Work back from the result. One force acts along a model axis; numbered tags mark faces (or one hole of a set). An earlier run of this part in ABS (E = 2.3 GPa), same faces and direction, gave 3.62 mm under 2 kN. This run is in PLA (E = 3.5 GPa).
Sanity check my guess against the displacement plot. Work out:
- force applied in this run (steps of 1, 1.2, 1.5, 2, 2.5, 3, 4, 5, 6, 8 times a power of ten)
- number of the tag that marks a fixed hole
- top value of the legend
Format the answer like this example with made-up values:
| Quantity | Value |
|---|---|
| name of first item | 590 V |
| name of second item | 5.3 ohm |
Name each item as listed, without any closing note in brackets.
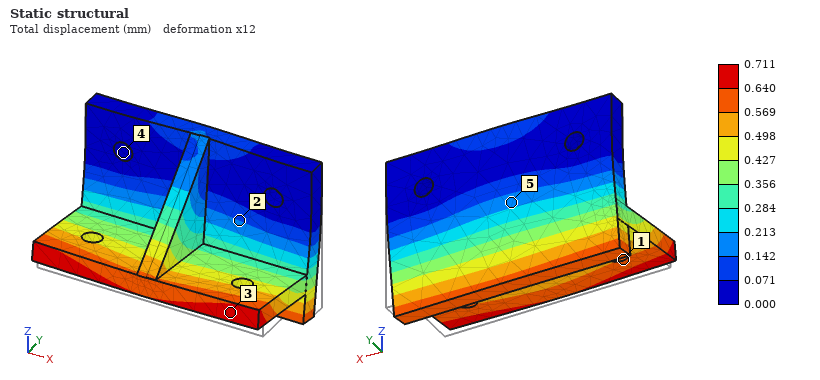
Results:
| Quantity | Value |
|---|---|
| force applied in this run | 600 N |
| number of the tag that marks a fixed hole | 4 |
| top value of the legend | 0.711 mm |
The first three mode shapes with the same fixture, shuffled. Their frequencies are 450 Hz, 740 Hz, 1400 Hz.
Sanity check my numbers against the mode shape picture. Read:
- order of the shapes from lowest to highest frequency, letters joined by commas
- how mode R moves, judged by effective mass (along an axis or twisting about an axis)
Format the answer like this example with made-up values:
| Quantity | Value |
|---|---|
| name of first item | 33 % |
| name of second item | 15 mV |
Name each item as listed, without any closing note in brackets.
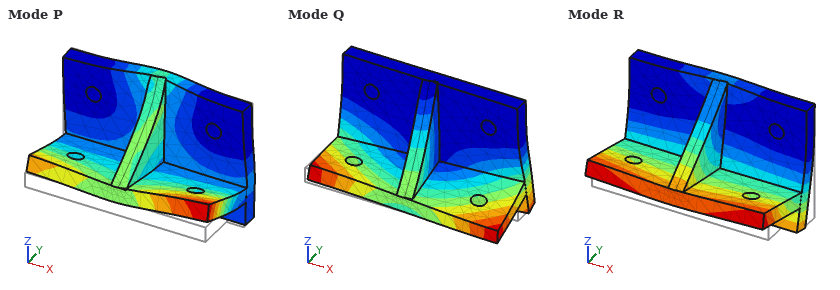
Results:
| Quantity | Value |
|---|---|
| order of the shapes from lowest to highest frequency, letters joined by commas | R, Q, P |
| how mode R moves, judged by effective mass | along Y |
